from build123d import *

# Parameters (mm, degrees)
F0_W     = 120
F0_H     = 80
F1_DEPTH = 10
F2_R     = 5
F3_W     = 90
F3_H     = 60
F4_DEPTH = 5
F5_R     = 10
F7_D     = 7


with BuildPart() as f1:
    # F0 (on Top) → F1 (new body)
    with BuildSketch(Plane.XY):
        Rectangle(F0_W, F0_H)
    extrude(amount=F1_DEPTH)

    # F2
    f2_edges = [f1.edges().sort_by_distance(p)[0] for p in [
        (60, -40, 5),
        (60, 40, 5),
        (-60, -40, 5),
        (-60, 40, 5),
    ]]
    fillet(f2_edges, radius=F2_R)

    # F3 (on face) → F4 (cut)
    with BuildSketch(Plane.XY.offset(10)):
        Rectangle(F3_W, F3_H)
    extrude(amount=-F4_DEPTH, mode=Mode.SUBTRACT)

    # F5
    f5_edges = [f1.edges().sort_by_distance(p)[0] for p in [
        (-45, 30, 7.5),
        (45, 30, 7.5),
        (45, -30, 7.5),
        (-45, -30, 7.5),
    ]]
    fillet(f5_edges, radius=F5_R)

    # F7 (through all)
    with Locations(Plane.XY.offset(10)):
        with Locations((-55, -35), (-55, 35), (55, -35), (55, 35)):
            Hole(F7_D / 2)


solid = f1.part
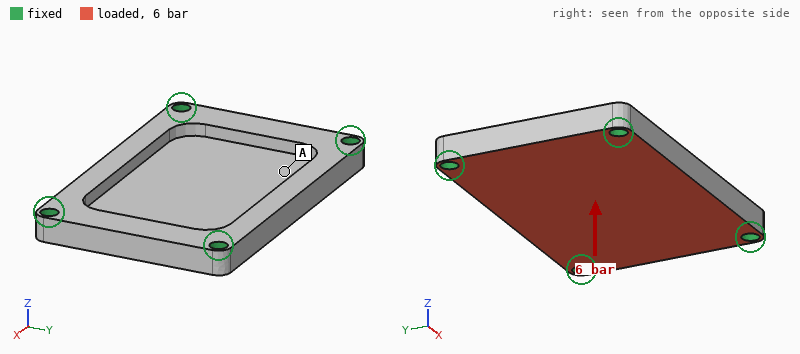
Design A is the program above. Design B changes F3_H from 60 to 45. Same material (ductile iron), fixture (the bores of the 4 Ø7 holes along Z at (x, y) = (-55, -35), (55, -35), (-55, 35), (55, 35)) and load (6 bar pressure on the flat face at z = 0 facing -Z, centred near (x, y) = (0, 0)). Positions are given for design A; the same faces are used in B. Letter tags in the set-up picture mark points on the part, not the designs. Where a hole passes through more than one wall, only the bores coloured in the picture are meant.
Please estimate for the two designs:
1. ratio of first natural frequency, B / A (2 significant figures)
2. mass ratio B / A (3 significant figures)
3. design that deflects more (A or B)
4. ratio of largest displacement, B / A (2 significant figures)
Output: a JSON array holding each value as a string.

["1.0", "1.10", "A", "0.81"]
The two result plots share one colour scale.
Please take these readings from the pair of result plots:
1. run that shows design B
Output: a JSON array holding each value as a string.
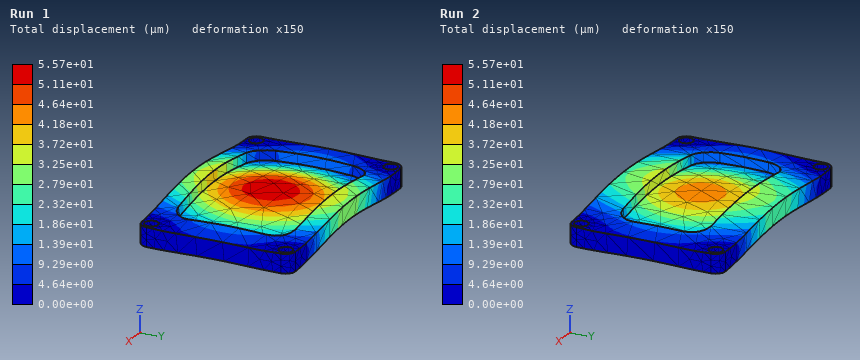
["Run 2"]
